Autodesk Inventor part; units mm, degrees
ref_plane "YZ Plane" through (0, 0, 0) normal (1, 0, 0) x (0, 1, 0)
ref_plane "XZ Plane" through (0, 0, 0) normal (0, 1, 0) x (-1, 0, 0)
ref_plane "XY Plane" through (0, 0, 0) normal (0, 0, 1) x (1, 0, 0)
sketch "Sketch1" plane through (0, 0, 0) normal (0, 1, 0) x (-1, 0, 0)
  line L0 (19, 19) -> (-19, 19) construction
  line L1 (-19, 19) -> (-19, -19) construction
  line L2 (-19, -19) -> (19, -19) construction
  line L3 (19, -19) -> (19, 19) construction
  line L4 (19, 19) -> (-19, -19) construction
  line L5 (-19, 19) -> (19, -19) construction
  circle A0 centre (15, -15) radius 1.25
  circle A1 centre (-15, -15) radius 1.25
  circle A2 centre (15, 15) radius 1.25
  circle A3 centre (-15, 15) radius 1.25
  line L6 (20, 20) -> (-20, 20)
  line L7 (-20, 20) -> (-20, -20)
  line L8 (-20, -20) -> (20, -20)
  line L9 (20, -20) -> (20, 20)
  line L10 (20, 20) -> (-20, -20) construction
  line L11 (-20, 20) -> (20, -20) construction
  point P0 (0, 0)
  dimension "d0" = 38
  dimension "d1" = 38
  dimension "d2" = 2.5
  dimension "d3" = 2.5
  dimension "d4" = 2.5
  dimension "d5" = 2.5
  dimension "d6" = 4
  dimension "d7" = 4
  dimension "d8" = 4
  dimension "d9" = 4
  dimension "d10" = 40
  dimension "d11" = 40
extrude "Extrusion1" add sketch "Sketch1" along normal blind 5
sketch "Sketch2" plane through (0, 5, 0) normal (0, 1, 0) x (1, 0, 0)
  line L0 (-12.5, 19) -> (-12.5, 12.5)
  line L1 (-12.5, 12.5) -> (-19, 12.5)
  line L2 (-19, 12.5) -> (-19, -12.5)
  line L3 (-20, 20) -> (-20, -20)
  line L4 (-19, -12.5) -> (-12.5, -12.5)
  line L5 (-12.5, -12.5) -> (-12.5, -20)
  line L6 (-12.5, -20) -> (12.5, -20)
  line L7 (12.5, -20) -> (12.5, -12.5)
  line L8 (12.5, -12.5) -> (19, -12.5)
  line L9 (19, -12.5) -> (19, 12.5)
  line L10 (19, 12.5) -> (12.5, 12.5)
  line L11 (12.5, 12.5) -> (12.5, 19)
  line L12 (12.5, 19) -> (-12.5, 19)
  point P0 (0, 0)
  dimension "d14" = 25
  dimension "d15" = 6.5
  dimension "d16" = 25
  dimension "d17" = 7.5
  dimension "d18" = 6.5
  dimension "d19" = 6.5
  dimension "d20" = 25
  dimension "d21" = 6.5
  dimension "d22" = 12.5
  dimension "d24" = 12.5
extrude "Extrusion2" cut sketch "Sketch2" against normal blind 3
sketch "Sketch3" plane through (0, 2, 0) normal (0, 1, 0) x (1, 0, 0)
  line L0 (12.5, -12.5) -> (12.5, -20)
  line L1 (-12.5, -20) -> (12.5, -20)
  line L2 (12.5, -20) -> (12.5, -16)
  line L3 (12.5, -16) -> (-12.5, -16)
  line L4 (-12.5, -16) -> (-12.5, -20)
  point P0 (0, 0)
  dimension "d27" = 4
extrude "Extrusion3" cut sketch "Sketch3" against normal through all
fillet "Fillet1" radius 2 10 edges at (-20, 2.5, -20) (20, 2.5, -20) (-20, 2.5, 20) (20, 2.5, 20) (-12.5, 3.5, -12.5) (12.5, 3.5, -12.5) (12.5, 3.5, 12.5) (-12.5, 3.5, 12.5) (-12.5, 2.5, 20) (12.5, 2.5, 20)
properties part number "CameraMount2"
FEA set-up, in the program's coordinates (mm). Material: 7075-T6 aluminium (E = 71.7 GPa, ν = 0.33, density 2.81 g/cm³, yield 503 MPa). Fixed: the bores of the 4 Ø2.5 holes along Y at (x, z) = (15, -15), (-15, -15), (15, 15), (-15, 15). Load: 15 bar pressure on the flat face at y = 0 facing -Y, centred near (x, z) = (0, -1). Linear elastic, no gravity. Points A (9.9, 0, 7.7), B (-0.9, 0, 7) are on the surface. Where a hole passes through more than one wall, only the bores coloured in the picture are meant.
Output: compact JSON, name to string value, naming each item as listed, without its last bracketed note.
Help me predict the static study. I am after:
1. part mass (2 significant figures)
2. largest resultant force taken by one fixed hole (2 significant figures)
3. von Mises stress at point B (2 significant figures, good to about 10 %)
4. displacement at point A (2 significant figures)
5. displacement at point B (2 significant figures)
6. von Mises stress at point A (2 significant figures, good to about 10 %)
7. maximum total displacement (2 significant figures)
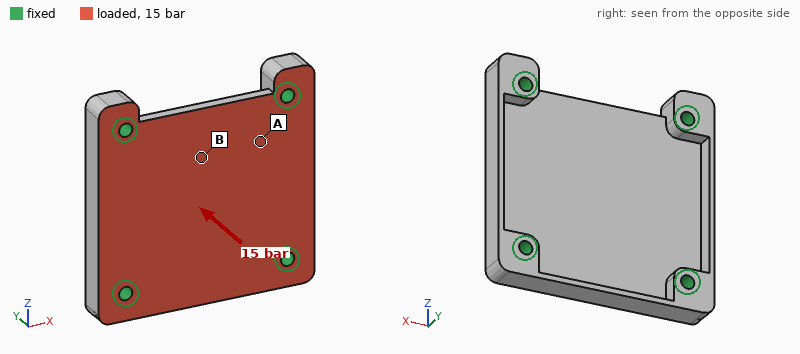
{"part mass": "11 g", "largest resultant force taken by one fixed hole": "610 N", "von Mises stress at point B": "90 MPa", "displacement at point A": "0.060 mm", "displacement at point B": "0.11 mm", "von Mises stress at point A": "36 MPa", "maximum total displacement": "0.12 mm"}
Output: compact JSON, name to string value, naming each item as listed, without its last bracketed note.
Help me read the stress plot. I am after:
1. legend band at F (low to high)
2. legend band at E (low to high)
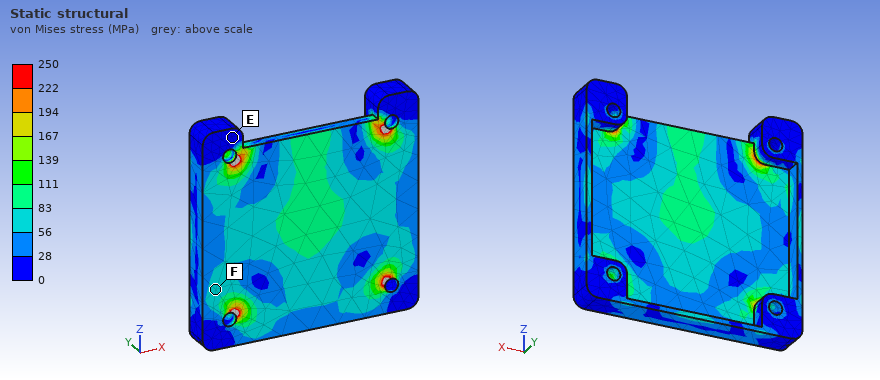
{"legend band at F": "56 to 83 MPa", "legend band at E": "0 to 28 MPa"}
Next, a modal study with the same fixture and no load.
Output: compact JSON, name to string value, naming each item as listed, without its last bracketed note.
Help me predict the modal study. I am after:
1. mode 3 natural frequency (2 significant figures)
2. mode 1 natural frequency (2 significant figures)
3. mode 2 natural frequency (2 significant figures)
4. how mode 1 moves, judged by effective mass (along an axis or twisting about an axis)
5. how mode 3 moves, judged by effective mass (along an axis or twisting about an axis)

{"mode 3 natural frequency": "18 kHz", "mode 1 natural frequency": "9100 Hz", "mode 2 natural frequency": "16 kHz", "how mode 1 moves, judged by effective mass": "along Y", "how mode 3 moves, judged by effective mass": "twisting about Z"}
